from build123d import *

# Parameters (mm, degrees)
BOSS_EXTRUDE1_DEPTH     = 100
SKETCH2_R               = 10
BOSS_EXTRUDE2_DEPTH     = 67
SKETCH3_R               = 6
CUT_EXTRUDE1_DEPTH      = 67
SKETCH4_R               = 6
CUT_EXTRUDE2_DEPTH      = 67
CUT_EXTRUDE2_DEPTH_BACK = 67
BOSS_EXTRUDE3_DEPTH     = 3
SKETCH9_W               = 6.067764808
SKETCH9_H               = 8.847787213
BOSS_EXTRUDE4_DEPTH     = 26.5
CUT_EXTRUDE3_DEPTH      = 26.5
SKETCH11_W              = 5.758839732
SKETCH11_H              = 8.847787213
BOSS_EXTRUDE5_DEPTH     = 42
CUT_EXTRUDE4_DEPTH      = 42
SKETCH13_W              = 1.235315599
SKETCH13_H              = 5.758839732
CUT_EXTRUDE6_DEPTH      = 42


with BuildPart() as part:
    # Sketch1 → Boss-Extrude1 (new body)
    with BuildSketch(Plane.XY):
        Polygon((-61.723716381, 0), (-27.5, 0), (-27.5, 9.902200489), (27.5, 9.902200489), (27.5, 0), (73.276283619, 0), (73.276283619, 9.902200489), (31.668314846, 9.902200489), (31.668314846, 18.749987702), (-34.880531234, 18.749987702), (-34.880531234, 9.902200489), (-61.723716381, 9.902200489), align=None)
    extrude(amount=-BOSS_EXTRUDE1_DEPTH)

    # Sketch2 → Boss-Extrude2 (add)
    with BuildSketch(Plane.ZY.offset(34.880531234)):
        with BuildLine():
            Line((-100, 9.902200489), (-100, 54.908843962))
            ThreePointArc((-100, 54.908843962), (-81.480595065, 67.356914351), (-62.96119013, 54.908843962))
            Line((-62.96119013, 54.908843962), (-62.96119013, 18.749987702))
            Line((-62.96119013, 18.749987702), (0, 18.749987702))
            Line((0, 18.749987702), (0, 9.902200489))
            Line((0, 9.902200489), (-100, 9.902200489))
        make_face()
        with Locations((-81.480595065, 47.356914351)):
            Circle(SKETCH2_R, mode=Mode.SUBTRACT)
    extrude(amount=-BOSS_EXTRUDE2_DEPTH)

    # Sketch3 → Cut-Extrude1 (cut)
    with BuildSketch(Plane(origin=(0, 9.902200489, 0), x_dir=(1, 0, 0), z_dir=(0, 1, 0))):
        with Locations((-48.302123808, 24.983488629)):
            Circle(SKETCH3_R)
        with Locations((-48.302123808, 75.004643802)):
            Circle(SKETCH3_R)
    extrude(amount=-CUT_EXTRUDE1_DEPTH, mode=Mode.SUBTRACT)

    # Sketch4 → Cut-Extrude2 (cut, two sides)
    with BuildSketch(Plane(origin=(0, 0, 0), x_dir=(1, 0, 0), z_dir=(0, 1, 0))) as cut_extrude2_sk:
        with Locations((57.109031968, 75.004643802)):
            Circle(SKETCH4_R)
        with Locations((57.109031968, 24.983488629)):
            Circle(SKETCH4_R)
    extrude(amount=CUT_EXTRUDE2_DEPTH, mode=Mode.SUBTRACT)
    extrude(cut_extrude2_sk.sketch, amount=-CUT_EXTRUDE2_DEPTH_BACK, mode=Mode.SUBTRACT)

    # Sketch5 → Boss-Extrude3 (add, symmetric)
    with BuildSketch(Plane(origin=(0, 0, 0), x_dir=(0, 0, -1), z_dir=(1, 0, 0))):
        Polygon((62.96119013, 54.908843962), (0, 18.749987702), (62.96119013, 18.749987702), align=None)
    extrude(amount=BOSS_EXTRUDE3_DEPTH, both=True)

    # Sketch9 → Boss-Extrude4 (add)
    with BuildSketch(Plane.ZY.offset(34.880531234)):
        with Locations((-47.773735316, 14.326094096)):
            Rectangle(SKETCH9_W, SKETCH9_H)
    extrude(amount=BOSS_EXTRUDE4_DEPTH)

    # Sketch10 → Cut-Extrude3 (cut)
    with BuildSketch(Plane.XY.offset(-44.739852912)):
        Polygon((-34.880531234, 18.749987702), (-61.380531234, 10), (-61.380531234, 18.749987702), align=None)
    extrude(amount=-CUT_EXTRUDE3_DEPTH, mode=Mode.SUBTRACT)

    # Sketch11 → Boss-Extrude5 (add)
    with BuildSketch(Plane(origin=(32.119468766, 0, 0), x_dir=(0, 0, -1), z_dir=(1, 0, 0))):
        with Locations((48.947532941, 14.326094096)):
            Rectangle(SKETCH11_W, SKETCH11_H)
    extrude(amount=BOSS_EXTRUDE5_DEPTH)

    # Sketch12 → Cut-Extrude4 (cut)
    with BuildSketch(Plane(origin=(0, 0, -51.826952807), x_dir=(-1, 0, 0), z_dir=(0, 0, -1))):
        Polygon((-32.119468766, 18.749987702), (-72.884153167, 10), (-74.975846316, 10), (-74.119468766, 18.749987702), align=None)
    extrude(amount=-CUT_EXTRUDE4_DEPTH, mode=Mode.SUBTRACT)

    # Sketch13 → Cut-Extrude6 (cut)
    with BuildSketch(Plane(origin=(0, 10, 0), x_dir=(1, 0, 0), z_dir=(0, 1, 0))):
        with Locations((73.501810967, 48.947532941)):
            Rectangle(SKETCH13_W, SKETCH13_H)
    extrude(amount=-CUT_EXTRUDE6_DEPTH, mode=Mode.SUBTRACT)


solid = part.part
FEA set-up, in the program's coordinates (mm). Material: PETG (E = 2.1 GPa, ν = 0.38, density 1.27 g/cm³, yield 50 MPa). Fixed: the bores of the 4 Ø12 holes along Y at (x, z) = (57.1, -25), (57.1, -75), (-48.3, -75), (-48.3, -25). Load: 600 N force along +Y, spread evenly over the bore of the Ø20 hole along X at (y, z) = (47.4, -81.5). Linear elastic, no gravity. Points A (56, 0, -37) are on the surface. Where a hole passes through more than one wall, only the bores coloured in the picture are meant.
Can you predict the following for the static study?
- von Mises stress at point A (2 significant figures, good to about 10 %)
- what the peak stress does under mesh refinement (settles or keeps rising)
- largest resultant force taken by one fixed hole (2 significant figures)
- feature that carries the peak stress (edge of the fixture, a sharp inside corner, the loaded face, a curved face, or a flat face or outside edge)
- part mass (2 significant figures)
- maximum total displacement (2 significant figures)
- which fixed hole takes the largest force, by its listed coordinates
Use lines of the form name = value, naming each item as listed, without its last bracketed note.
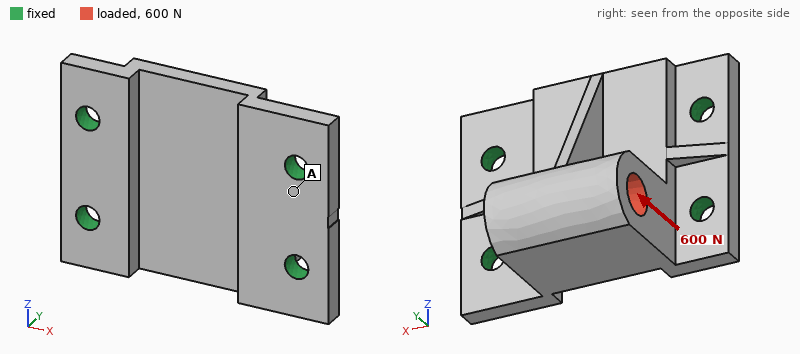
von Mises stress at point A = 0.92 MPa
what the peak stress does under mesh refinement = keeps rising
largest resultant force taken by one fixed hole = 470 N
feature that carries the peak stress = edge of the fixture
part mass = 300 g
maximum total displacement = 0.18 mm
which fixed hole takes the largest force, by its listed coordinates = (-48.3, -75)
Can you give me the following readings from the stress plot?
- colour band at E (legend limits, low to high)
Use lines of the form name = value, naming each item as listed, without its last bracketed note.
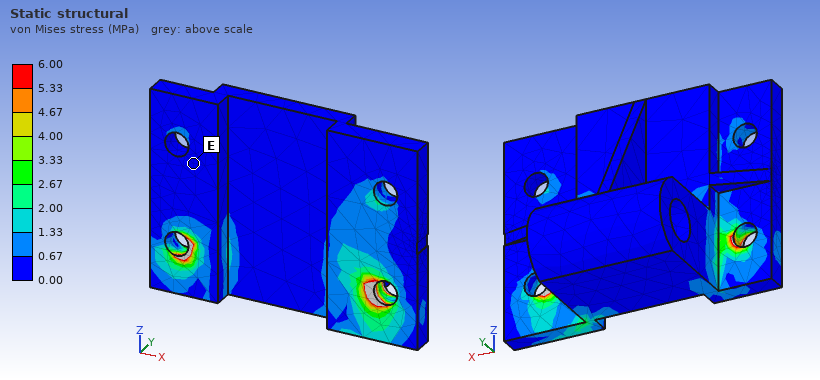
colour band at E = 0.00 to 0.67 MPa
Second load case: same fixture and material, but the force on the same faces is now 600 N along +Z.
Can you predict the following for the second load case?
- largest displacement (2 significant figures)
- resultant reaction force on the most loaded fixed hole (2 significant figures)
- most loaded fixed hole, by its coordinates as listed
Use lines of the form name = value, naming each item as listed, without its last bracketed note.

largest displacement = 0.32 mm
resultant reaction force on the most loaded fixed hole = 520 N
most loaded fixed hole, by its coordinates as listed = (-48.3, -25)
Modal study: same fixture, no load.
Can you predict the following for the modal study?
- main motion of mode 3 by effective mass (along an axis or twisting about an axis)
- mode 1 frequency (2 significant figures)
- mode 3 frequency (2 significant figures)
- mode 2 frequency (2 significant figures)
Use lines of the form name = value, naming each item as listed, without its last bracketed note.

main motion of mode 3 by effective mass = along Y
mode 1 frequency = 720 Hz
mode 3 frequency = 1500 Hz
mode 2 frequency = 1000 Hz
